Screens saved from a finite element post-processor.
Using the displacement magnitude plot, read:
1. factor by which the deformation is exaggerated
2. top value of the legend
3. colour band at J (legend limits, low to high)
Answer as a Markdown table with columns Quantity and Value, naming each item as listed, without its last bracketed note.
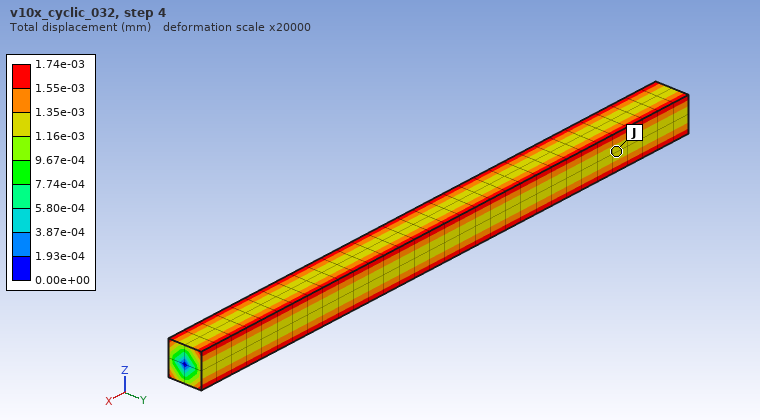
| Quantity | Value |
|---|---|
| factor by which the deformation is exaggerated | 20000 |
| top value of the legend | 1.74e-03 mm |
| colour band at J | 1.16e-03 to 1.35e-03 mm |
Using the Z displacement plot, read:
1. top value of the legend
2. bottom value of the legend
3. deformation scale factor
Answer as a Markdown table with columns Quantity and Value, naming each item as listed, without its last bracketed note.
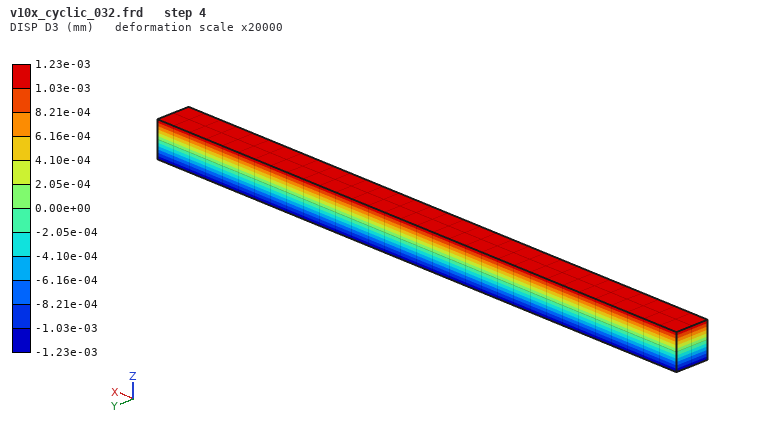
| Quantity | Value |
|---|---|
| top value of the legend | 1.23e-03 mm |
| bottom value of the legend | -1.23e-03 mm |
| deformation scale factor | 20000 |
